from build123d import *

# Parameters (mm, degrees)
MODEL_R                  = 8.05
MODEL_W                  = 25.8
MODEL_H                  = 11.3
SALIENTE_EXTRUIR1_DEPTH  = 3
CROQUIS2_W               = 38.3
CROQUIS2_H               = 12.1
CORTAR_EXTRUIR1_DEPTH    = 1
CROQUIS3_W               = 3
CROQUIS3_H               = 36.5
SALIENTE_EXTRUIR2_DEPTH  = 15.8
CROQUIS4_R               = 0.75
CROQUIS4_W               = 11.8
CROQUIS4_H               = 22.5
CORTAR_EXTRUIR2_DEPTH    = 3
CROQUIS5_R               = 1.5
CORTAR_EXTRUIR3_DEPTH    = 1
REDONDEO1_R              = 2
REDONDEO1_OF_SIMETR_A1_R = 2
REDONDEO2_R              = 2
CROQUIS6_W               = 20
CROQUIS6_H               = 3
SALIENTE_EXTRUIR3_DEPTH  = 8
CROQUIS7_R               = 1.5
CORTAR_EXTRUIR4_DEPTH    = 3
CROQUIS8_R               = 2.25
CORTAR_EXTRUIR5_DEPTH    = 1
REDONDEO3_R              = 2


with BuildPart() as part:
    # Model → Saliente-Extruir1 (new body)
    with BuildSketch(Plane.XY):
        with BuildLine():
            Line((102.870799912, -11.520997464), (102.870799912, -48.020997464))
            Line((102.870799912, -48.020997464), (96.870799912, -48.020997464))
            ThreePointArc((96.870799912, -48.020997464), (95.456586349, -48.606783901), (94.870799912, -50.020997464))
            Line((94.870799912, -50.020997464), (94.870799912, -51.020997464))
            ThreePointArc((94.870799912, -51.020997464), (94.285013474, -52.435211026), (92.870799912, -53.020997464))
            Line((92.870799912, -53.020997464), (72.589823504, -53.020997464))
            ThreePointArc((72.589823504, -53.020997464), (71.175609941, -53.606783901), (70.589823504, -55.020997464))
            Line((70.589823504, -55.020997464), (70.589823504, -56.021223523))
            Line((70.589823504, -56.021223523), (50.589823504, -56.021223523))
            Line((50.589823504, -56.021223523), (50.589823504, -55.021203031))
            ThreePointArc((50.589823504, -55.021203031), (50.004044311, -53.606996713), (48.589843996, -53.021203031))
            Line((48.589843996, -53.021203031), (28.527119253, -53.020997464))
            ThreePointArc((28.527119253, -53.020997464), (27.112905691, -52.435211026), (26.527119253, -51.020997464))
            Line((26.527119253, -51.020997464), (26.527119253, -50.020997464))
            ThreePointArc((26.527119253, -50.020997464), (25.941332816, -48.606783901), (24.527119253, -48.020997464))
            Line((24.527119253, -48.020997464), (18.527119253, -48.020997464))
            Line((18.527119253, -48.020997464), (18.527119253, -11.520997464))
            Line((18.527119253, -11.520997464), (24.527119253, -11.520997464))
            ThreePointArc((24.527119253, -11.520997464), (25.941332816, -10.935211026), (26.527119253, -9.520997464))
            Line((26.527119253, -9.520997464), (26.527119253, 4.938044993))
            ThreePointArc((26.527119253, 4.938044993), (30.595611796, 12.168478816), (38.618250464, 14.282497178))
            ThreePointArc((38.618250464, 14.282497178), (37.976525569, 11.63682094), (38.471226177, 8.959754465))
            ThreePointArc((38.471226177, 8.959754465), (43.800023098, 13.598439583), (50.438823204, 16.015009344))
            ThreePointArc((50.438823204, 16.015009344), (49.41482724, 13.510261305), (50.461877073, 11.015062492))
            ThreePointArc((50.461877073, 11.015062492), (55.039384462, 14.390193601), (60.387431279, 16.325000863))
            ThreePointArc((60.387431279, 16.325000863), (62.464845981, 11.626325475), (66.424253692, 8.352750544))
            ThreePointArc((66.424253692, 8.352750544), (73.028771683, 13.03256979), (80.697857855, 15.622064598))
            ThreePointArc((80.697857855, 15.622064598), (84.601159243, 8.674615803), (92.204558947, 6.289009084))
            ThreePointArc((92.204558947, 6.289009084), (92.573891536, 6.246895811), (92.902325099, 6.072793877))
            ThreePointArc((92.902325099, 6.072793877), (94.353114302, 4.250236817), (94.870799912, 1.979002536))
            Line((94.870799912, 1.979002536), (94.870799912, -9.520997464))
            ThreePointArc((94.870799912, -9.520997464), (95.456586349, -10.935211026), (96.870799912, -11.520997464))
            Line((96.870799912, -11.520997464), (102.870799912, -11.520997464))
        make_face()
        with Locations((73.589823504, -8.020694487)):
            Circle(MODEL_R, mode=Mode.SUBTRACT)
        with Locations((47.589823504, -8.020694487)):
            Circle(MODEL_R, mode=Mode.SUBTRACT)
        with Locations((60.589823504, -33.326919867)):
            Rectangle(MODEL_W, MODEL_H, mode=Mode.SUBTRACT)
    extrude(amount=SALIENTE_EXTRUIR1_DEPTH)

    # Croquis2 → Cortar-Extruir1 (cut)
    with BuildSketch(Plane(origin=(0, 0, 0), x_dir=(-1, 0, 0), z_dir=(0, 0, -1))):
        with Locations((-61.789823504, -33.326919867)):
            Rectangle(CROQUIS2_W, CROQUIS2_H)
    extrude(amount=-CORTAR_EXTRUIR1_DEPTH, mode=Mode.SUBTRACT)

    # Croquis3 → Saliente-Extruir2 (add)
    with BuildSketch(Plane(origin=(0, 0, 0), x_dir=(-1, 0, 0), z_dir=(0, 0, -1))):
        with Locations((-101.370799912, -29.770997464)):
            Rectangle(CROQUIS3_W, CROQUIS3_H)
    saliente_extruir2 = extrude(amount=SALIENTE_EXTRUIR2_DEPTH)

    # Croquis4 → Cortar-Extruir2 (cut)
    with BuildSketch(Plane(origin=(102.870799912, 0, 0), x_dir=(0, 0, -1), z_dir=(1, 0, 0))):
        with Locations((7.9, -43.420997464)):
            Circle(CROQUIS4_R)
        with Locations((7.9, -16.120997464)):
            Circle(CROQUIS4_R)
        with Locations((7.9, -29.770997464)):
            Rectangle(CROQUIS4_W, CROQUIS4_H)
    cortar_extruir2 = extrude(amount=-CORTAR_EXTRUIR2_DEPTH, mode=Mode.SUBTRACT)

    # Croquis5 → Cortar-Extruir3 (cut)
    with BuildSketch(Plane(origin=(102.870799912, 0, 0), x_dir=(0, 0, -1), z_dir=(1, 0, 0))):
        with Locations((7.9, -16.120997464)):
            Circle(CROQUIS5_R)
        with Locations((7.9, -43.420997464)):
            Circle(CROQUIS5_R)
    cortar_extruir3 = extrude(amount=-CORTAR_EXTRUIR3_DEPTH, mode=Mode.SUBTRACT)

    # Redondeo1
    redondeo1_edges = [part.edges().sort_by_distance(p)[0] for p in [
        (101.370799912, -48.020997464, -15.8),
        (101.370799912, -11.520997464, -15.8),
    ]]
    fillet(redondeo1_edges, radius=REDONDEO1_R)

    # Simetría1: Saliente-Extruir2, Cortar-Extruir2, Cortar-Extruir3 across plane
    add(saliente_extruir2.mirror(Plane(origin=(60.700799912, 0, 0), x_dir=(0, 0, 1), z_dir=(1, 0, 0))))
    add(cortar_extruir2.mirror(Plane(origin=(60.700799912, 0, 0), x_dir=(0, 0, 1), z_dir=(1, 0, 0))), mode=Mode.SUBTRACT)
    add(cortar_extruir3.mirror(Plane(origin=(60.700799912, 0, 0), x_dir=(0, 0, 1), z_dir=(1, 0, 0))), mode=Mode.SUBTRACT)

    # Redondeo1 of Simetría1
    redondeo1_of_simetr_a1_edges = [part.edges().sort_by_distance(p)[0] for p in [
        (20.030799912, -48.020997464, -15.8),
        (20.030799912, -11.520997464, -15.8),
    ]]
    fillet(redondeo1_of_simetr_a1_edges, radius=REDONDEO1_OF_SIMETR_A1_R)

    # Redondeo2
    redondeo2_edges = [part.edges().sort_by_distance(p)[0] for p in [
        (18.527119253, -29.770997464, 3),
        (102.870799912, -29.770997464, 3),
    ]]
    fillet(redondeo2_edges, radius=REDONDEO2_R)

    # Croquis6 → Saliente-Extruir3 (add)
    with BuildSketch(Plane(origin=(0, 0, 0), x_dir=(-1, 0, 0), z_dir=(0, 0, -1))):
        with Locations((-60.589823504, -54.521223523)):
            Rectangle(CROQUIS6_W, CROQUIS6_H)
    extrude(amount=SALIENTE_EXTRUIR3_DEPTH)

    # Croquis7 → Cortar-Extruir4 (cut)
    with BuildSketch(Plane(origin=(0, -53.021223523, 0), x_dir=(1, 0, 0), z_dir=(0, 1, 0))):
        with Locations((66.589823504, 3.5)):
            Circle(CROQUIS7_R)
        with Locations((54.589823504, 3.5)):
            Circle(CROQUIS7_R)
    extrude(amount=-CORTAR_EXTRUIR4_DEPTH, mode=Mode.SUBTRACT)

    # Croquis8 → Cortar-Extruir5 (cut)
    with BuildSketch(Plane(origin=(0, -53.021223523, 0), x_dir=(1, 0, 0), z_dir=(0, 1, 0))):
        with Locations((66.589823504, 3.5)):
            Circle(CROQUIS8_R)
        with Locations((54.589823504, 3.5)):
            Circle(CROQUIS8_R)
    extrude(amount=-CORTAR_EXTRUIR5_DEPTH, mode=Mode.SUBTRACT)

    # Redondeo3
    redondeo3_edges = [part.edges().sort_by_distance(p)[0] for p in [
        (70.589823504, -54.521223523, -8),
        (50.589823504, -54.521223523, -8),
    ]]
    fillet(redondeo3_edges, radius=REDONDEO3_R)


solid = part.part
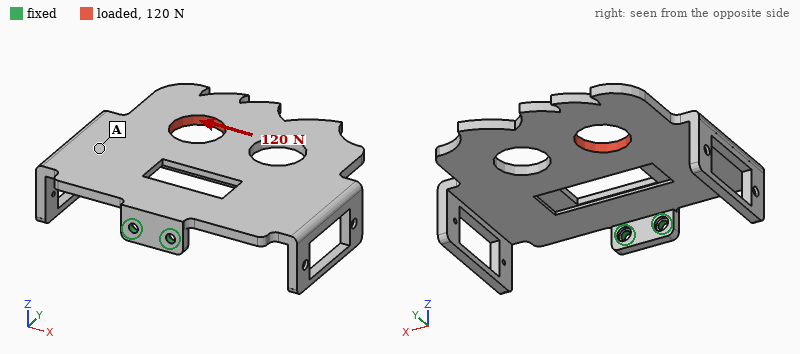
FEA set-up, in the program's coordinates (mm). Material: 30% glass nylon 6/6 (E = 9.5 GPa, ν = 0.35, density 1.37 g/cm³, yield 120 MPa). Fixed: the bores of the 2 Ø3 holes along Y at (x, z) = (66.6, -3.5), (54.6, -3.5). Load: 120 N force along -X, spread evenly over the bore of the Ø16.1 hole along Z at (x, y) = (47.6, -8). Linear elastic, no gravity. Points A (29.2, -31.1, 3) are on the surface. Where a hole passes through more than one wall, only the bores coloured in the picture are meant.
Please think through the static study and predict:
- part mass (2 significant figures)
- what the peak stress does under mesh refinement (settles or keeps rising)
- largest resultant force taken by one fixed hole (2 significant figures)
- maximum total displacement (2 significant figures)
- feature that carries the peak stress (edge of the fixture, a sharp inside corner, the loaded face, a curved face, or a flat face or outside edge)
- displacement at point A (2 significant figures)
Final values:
21 g
keeps rising
420 N
1.1 mm
edge of the fixture
0.65 mm
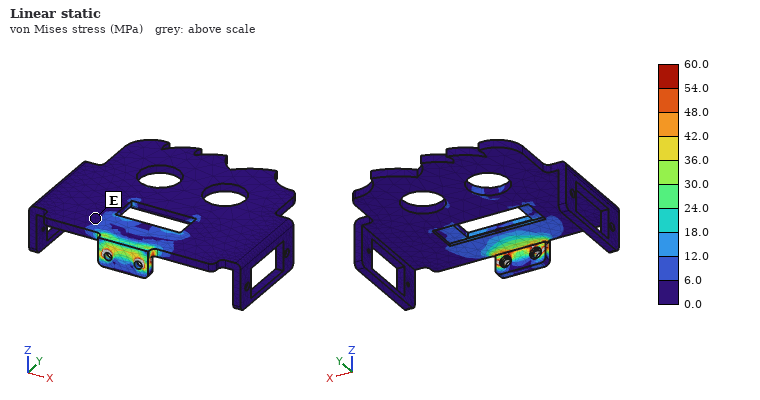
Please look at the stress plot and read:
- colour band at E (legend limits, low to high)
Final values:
0.0 to 6.0 MPa
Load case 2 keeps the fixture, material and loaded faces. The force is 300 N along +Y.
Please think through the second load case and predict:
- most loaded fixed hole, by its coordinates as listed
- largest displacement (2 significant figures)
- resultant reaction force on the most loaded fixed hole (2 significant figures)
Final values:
(54.6, -3.5)
1.3 mm
440 N
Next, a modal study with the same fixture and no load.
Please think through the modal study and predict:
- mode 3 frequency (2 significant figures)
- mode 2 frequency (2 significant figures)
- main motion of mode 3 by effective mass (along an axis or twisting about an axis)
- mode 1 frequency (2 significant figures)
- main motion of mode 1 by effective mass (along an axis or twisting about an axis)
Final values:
510 Hz
280 Hz
along X
160 Hz
along Z
